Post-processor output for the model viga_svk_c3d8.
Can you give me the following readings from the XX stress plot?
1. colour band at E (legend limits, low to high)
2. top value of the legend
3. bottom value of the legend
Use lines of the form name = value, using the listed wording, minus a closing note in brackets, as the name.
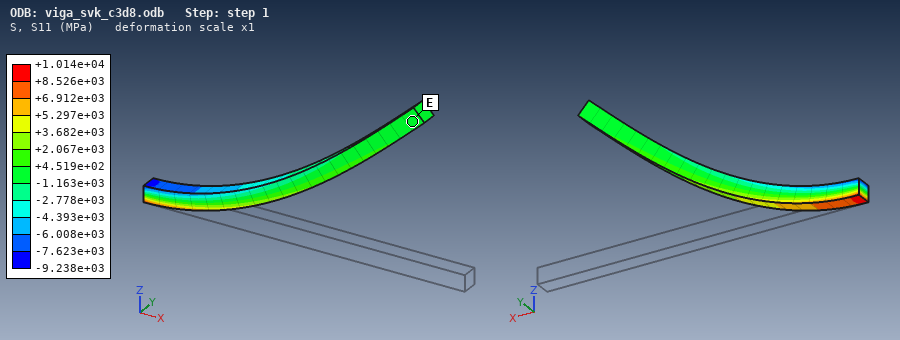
colour band at E = -1.163e+03 to +4.519e+02 MPa
top value of the legend = +1.014e+04 MPa
bottom value of the legend = -9.238e+03 MPa
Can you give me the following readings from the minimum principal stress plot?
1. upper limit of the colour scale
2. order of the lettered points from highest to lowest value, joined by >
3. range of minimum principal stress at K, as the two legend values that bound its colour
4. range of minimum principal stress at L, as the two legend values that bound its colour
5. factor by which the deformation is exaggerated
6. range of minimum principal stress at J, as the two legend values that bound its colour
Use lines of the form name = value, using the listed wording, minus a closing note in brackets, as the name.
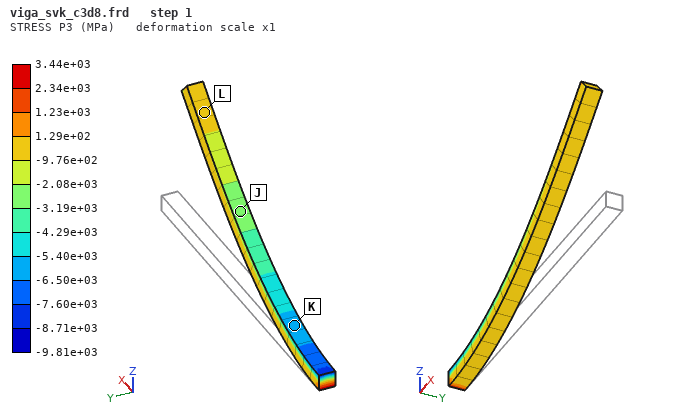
upper limit of the colour scale = 3.44e+03 MPa
order of the lettered points from highest to lowest value, joined by > = L > J > K
range of minimum principal stress at K, as the two legend values that bound its colour = -6.50e+03 to -5.40e+03 MPa
range of minimum principal stress at L, as the two legend values that bound its colour = -9.76e+02 to 1.29e+02 MPa
factor by which the deformation is exaggerated = 1
range of minimum principal stress at J, as the two legend values that bound its colour = -3.19e+03 to -2.08e+03 MPa
